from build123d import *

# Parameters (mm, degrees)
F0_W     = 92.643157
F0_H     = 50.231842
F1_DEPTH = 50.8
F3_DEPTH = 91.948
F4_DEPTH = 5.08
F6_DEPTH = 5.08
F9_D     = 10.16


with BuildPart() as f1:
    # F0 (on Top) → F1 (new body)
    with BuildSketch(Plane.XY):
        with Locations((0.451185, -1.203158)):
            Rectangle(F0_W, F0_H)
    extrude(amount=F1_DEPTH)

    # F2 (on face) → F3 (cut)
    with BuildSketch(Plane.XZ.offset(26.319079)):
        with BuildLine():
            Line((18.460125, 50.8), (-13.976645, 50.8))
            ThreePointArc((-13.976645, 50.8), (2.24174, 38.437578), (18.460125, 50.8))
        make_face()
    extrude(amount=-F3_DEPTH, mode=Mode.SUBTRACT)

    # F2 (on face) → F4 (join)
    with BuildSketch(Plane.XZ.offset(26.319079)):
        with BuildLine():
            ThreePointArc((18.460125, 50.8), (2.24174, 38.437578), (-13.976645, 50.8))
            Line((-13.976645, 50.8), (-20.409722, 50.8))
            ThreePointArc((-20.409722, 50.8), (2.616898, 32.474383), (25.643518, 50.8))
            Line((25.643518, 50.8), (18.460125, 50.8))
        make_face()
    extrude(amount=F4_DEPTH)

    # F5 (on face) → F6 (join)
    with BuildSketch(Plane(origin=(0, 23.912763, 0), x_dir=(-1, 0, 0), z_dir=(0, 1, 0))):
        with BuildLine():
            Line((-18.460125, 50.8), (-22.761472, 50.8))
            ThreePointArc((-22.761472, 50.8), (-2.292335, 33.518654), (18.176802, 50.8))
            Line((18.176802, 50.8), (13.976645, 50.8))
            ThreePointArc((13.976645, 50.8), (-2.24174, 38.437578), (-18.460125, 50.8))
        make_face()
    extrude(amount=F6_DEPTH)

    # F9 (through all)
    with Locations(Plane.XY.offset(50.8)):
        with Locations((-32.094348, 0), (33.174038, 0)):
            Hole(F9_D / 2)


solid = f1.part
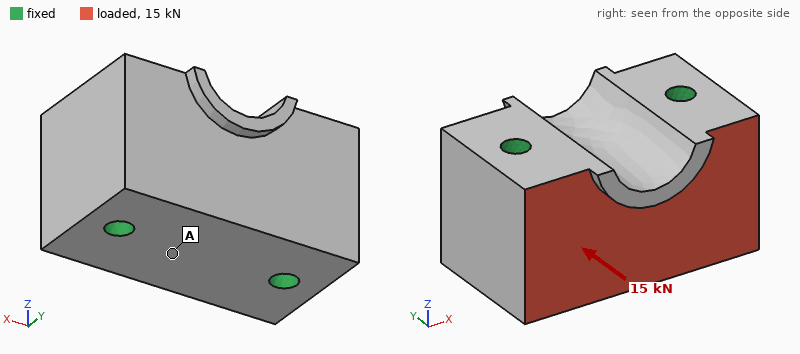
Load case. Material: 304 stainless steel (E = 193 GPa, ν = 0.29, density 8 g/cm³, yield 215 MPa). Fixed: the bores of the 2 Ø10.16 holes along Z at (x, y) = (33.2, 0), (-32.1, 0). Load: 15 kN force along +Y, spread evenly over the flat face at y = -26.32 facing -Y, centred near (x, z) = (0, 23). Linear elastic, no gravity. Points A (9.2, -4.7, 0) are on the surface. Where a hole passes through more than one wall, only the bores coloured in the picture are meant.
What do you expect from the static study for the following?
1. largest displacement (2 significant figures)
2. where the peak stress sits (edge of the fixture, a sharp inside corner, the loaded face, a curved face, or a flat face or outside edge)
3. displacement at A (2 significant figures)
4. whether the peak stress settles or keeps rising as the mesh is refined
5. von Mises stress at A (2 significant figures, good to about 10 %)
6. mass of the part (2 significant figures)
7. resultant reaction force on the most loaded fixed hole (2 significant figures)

1.2 µm
edge of the fixture
0.81 µm
keeps rising
2.4 MPa
1.7 kg
7.6 kN
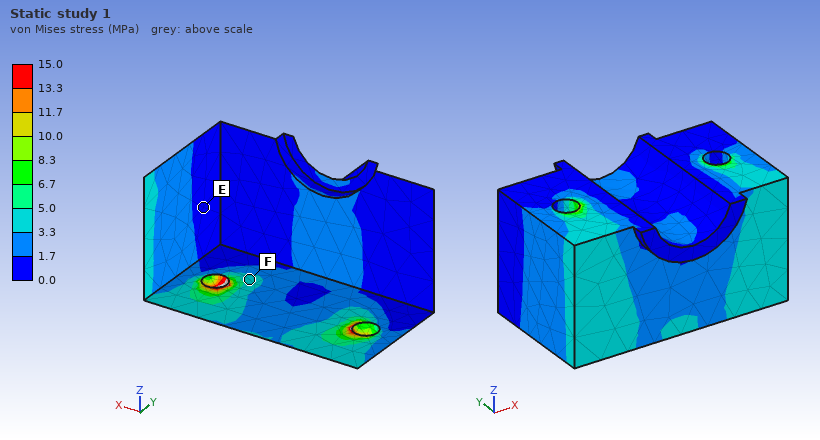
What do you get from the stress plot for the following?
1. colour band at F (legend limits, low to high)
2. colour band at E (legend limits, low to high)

3.3 to 5.0 MPa
0.0 to 1.7 MPa
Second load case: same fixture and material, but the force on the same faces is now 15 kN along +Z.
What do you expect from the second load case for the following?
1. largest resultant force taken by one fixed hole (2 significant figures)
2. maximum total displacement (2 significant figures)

7.6 kN
3.6 µm
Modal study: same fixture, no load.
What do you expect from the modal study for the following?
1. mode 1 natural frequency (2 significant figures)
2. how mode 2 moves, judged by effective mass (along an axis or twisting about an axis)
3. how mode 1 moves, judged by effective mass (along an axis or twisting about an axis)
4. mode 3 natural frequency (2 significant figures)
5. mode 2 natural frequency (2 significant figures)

17 kHz
along Z
along Y
20 kHz
18 kHz
